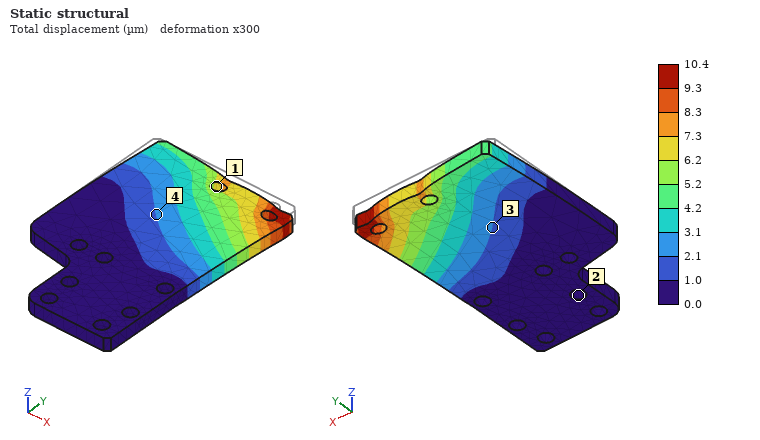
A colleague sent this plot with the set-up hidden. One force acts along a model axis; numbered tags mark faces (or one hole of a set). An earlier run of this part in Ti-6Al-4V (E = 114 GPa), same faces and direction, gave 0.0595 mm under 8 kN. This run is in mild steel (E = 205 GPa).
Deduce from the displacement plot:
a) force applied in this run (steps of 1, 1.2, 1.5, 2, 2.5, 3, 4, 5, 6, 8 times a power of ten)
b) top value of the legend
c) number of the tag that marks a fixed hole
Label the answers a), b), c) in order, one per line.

a) 2.5 kN
b) 10.4 µm
c) 2
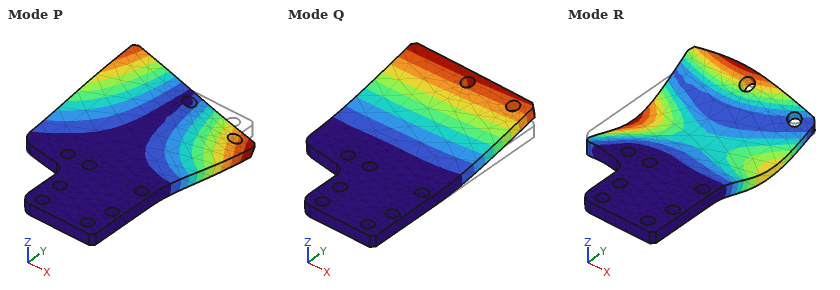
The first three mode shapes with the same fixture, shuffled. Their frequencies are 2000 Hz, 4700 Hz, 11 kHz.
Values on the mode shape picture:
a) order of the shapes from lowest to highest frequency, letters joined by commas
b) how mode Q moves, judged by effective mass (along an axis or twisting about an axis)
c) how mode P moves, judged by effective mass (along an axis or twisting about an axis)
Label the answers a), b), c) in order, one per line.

a) Q, P, R
b) along Z
c) twisting about Y
